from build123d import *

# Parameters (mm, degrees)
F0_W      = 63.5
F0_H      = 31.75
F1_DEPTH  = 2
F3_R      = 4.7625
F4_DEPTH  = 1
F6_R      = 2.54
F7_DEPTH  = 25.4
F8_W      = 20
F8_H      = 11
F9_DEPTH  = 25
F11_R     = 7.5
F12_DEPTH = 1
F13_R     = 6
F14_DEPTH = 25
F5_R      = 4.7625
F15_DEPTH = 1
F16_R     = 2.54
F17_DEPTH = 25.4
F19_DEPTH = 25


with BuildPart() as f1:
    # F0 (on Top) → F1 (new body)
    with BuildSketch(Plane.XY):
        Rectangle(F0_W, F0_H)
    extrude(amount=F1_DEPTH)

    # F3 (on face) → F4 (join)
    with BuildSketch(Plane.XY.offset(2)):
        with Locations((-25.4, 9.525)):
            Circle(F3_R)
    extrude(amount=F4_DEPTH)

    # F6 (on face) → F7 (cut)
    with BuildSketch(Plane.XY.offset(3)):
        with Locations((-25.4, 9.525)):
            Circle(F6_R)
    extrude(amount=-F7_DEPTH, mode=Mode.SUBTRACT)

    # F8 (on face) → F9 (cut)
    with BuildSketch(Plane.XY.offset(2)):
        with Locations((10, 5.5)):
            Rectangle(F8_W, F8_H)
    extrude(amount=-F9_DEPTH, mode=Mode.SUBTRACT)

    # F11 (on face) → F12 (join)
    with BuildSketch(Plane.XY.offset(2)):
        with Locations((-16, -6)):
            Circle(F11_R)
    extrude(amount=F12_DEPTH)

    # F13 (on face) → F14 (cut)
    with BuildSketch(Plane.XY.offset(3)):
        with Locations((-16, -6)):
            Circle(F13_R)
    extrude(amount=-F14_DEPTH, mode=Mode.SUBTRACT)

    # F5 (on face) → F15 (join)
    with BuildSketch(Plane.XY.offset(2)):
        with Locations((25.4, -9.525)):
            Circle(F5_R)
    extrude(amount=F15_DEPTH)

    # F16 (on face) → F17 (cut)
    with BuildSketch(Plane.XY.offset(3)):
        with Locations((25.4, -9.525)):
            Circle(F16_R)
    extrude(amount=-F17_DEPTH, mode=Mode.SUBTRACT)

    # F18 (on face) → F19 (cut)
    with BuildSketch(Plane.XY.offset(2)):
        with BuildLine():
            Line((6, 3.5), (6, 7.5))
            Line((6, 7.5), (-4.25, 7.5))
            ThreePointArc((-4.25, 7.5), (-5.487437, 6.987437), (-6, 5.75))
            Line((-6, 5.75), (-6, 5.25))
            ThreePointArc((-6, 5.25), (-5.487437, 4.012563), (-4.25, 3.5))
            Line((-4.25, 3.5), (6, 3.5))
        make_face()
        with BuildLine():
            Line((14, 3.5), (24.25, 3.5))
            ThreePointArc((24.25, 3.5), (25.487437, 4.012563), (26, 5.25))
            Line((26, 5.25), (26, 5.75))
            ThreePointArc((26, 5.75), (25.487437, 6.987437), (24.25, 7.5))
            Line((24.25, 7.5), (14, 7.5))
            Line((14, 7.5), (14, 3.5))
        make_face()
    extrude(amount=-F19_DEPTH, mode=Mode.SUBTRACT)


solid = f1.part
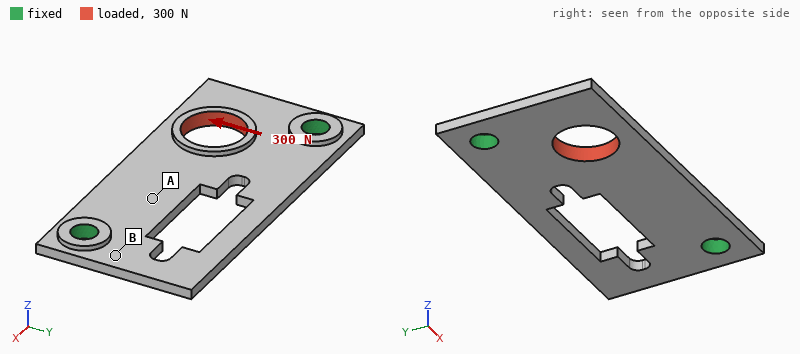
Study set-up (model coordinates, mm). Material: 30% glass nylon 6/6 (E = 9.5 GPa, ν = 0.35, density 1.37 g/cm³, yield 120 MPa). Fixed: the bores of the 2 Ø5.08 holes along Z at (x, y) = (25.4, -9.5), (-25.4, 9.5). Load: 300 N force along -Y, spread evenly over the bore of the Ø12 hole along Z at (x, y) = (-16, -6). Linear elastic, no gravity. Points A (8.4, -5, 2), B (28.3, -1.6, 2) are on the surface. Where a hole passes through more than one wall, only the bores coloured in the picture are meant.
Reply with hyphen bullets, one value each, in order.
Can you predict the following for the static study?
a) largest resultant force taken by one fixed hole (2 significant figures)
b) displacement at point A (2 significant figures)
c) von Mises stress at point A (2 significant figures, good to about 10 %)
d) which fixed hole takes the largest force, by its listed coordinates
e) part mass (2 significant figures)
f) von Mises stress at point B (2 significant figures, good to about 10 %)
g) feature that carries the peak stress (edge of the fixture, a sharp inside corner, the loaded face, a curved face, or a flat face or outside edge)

- 270 N
- 0.024 mm
- 5.4 MPa
- (-25.4, 9.5)
- 4.6 g
- 2.2 MPa
- edge of the fixture
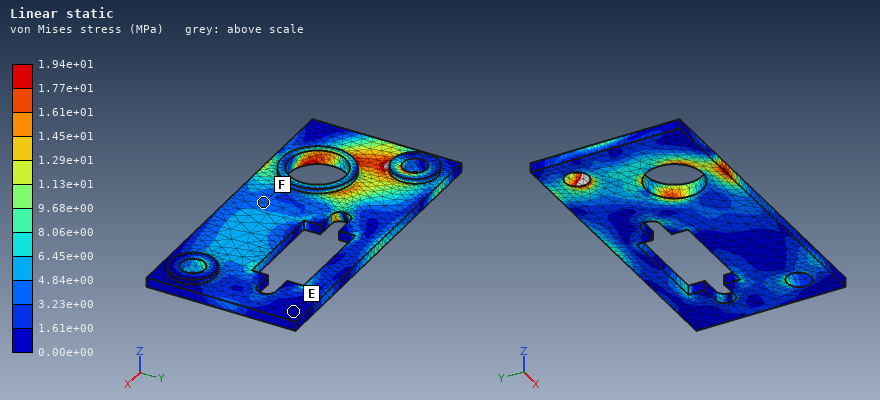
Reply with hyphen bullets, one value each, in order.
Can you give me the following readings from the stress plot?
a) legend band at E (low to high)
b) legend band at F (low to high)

- 0.00e+00 to 1.61e+00 MPa
- 3.23e+00 to 4.84e+00 MPa
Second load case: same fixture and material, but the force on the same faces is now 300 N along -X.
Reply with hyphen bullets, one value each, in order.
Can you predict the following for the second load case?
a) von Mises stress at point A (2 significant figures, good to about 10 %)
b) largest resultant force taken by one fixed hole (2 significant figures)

- 5.2 MPa
- 150 N
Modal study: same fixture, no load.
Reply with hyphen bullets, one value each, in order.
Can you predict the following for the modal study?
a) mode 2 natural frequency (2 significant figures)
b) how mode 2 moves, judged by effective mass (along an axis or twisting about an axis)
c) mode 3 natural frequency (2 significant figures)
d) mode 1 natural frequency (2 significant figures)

- 1600 Hz
- along Z
- 2500 Hz
- 1500 Hz
